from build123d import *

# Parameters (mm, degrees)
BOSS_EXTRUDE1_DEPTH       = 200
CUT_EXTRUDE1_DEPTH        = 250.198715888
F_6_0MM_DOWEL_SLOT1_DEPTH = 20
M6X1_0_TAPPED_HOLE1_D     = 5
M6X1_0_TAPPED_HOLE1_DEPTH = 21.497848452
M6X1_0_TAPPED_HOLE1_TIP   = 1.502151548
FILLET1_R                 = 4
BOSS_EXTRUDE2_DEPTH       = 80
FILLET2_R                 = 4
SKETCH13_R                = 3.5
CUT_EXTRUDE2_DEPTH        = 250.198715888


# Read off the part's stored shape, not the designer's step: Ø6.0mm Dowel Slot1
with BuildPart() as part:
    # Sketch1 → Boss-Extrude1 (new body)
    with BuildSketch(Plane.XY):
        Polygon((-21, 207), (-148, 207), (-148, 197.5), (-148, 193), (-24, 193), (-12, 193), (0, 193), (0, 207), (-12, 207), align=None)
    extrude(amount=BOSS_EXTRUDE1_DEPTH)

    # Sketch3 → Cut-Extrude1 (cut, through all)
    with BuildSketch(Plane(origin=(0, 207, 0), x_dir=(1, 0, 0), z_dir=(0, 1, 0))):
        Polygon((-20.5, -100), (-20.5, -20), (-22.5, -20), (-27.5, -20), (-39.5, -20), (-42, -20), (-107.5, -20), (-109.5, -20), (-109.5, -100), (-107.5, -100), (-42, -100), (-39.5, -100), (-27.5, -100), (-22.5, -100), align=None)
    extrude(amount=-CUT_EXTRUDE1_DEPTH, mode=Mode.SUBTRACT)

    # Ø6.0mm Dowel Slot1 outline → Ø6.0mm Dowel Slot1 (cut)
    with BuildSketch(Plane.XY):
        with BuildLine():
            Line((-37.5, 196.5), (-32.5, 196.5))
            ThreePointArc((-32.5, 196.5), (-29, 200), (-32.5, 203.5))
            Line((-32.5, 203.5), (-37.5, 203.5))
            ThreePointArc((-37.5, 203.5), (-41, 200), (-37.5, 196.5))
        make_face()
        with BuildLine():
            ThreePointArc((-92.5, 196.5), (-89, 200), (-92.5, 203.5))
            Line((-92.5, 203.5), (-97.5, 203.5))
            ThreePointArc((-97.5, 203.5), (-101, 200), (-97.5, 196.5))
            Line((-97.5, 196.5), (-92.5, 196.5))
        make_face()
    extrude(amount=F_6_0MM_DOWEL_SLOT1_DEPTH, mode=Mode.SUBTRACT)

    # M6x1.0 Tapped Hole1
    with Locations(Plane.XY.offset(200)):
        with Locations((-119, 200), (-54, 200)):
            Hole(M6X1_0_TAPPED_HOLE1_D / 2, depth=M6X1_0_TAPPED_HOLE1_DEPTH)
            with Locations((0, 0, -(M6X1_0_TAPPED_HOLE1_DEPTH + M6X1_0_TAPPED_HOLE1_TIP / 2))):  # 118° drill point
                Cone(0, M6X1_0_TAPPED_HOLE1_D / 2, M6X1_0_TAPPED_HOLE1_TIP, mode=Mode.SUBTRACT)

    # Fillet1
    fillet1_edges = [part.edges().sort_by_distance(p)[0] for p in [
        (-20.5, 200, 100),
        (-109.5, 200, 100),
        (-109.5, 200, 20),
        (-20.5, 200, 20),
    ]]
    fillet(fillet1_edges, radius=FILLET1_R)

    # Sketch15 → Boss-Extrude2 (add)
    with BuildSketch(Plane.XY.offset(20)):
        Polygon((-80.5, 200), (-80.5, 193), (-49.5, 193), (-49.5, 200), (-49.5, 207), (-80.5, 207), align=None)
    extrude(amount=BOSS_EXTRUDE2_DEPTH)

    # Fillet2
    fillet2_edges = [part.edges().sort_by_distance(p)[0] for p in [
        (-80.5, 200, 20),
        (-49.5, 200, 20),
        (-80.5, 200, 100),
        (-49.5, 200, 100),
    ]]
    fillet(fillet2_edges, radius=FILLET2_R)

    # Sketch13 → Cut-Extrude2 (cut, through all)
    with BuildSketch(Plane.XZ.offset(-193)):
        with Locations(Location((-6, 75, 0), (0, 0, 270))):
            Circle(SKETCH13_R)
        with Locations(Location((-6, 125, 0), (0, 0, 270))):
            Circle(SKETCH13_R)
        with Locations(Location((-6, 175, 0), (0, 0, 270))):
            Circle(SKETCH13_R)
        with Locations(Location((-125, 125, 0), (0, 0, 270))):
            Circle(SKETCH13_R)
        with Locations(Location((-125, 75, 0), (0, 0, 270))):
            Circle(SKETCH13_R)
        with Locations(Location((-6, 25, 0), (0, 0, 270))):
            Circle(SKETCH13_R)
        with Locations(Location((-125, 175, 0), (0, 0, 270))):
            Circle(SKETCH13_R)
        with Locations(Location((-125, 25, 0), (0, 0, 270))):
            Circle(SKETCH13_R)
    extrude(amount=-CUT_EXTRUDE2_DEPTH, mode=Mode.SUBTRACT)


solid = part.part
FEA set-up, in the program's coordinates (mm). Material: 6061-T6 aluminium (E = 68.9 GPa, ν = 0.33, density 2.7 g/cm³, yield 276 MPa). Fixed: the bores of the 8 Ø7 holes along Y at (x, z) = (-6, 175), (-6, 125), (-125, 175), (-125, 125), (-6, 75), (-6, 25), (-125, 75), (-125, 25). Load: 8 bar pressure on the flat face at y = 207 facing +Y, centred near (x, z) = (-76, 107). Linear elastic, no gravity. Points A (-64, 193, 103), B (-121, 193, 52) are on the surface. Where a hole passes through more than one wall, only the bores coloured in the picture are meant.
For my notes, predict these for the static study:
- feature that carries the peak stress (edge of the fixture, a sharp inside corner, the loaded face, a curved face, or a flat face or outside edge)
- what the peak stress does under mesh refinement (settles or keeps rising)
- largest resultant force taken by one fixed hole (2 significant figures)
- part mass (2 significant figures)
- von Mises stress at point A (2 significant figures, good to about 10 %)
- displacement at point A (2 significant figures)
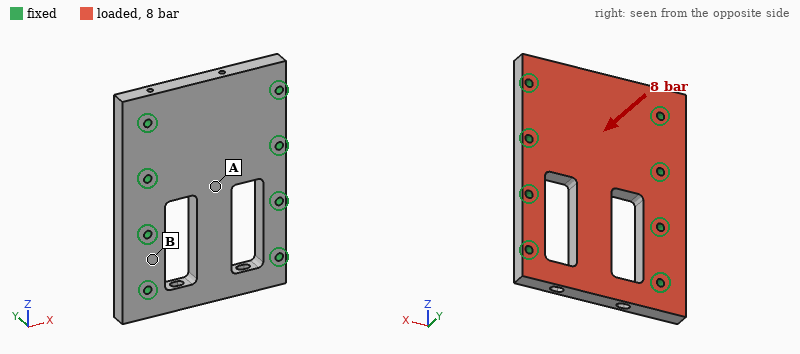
edge of the fixture
keeps rising
3.6 kN
920 g
21 MPa
60 µm
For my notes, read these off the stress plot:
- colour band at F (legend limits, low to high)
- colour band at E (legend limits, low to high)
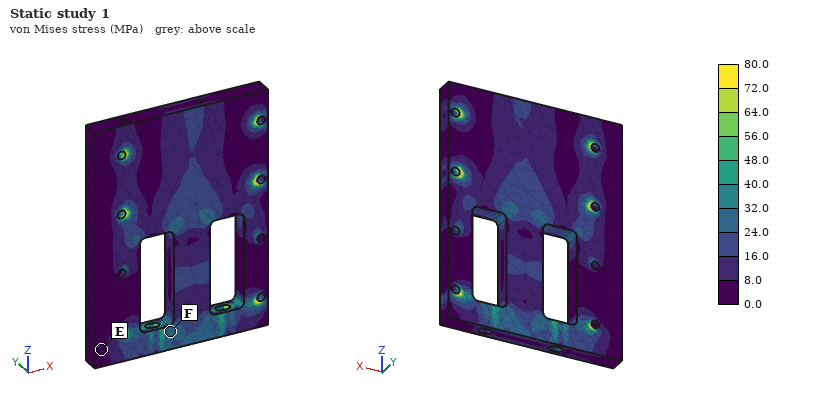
24.0 to 32.0 MPa
0.0 to 8.0 MPa
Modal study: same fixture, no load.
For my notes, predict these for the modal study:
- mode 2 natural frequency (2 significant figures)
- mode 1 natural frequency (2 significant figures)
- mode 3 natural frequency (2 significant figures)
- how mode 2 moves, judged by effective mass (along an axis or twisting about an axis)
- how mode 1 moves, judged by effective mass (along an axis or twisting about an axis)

4100 Hz
2800 Hz
4700 Hz
along Y
along Y
